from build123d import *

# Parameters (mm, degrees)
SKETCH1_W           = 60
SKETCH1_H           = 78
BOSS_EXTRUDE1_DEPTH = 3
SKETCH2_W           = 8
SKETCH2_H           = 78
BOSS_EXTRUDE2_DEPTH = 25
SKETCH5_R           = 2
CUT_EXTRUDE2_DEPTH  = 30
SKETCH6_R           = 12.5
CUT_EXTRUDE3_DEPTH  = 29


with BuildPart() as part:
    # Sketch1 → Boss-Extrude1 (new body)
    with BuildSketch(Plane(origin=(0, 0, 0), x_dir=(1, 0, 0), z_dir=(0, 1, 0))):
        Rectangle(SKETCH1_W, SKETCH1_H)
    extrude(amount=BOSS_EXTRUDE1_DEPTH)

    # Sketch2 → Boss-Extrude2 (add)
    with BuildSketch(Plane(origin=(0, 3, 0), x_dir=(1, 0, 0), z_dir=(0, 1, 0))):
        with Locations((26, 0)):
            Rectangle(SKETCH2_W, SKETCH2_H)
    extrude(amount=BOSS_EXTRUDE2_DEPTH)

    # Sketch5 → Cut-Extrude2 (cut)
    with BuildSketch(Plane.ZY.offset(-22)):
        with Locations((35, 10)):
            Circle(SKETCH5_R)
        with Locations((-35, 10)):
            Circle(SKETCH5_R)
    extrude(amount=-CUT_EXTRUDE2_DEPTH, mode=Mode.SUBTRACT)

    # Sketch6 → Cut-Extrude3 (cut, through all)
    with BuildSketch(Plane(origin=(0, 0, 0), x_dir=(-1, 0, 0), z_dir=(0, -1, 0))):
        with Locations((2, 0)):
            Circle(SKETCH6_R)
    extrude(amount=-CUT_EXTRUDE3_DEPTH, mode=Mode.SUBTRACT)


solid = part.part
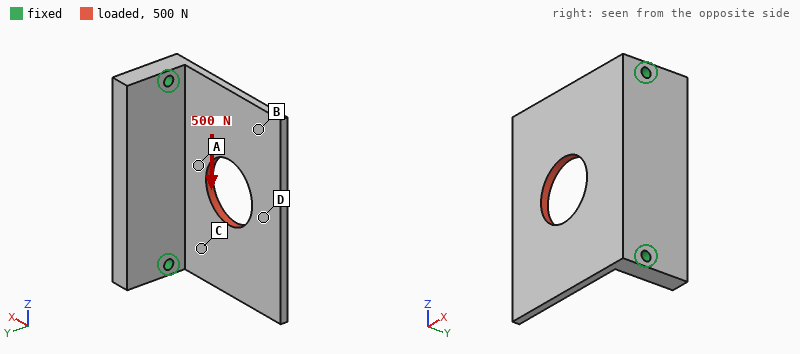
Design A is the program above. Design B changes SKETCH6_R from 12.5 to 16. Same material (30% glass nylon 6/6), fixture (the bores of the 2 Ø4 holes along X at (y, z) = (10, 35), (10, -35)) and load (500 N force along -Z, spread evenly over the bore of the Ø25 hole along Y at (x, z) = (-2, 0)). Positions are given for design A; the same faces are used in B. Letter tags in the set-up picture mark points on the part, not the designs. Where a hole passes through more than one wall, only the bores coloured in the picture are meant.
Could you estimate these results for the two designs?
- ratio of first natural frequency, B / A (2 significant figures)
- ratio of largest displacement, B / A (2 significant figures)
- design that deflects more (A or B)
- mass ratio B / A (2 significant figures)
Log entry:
0.96
1.2
B
0.97
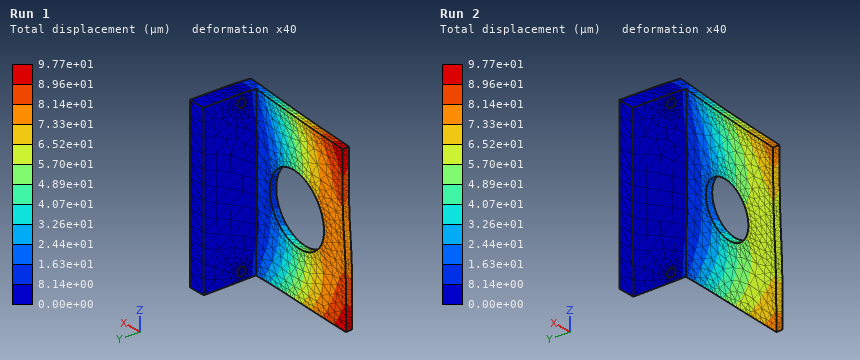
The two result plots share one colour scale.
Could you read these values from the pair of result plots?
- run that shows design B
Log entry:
Run 1
